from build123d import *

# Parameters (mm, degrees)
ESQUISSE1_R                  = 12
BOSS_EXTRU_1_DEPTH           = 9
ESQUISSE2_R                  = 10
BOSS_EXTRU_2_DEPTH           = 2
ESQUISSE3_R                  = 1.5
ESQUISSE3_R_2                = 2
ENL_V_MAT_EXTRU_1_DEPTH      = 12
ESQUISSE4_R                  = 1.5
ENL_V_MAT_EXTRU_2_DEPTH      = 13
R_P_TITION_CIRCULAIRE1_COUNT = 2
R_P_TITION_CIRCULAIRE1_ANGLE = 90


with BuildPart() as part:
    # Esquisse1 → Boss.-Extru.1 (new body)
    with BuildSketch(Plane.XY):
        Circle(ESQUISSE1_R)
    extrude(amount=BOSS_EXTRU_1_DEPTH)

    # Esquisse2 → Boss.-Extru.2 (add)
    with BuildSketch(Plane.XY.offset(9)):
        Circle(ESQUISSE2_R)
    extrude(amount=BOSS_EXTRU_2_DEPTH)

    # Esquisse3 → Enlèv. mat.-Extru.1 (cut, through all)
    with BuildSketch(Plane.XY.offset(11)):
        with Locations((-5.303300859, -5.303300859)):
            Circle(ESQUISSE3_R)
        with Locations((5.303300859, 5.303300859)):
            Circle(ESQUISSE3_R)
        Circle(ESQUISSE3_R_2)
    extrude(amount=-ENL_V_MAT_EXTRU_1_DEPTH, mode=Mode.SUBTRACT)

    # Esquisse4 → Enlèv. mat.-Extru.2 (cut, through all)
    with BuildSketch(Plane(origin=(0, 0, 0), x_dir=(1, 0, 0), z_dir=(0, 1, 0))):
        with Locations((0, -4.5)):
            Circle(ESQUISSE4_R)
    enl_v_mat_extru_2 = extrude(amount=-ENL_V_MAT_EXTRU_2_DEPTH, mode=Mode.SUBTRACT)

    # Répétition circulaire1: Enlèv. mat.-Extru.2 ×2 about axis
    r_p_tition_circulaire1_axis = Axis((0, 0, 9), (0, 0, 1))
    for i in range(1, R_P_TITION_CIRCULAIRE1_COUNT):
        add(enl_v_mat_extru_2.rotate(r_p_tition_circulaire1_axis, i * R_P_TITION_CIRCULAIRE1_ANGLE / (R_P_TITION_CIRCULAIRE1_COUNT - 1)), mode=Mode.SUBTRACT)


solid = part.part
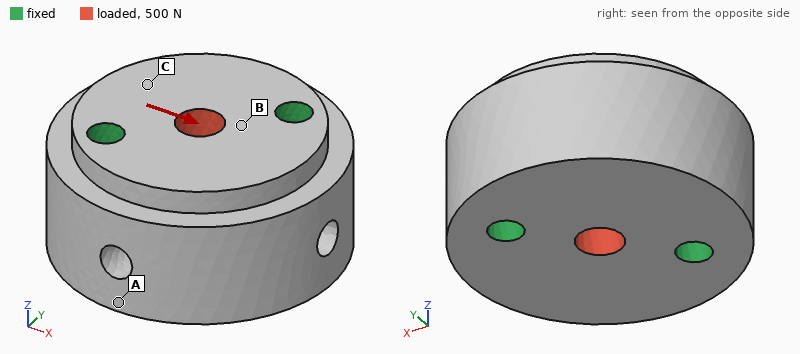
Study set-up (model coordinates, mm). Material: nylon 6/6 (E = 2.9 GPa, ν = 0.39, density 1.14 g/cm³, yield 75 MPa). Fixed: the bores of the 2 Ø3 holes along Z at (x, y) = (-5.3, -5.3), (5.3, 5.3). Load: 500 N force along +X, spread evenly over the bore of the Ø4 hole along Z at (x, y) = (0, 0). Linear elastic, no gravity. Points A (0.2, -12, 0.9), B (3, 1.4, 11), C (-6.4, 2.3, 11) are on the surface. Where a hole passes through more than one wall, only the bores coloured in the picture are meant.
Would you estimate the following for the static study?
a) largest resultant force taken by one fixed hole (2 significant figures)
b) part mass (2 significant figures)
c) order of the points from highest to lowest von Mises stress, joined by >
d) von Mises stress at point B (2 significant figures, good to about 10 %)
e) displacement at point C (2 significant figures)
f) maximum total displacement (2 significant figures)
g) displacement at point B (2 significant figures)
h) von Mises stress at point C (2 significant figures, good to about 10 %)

260 N
4.9 g
B > C > A
3.7 MPa
7.1 µm
11 µm
7.8 µm
1.5 MPa
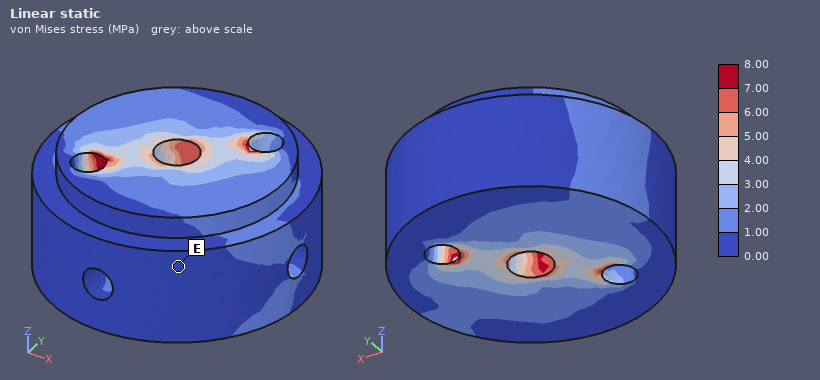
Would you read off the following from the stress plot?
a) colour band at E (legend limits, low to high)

0.00 to 1.00 MPa
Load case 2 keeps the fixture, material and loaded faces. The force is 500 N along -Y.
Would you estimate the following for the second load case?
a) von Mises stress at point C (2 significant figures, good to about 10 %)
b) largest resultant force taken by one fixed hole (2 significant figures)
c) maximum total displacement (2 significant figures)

1.5 MPa
260 N
11 µm
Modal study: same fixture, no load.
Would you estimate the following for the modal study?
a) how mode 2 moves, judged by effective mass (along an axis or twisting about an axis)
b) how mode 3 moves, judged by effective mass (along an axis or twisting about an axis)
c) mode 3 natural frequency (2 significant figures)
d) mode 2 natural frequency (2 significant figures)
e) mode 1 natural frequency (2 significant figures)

along Z
twisting about Z
20 kHz
15 kHz
13 kHz
